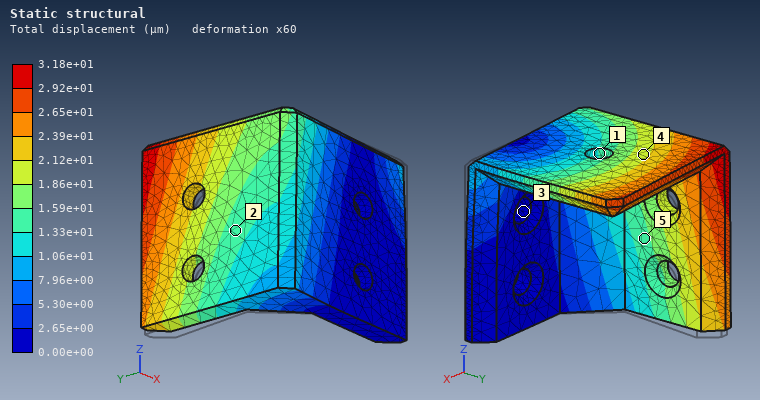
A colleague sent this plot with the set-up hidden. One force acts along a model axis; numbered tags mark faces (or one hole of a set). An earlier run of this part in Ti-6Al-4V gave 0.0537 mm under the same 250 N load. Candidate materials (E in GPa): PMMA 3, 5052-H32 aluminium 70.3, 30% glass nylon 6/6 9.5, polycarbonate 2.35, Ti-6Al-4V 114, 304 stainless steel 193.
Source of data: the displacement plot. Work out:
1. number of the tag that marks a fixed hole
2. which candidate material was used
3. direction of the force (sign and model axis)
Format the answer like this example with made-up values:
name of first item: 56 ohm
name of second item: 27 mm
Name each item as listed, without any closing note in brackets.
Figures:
number of the tag that marks a fixed hole: 3
which candidate material was used: 304 stainless steel
direction of the force: -X
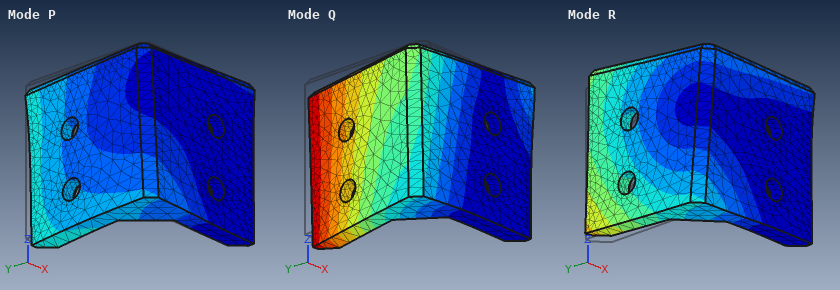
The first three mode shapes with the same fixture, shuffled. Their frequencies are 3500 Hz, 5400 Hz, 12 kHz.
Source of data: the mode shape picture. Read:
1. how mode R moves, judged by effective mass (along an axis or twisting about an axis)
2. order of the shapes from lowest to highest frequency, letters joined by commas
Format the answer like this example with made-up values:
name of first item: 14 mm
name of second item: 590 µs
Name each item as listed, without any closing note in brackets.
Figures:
how mode R moves, judged by effective mass: along Z
order of the shapes from lowest to highest frequency, letters joined by commas: Q, R, P
